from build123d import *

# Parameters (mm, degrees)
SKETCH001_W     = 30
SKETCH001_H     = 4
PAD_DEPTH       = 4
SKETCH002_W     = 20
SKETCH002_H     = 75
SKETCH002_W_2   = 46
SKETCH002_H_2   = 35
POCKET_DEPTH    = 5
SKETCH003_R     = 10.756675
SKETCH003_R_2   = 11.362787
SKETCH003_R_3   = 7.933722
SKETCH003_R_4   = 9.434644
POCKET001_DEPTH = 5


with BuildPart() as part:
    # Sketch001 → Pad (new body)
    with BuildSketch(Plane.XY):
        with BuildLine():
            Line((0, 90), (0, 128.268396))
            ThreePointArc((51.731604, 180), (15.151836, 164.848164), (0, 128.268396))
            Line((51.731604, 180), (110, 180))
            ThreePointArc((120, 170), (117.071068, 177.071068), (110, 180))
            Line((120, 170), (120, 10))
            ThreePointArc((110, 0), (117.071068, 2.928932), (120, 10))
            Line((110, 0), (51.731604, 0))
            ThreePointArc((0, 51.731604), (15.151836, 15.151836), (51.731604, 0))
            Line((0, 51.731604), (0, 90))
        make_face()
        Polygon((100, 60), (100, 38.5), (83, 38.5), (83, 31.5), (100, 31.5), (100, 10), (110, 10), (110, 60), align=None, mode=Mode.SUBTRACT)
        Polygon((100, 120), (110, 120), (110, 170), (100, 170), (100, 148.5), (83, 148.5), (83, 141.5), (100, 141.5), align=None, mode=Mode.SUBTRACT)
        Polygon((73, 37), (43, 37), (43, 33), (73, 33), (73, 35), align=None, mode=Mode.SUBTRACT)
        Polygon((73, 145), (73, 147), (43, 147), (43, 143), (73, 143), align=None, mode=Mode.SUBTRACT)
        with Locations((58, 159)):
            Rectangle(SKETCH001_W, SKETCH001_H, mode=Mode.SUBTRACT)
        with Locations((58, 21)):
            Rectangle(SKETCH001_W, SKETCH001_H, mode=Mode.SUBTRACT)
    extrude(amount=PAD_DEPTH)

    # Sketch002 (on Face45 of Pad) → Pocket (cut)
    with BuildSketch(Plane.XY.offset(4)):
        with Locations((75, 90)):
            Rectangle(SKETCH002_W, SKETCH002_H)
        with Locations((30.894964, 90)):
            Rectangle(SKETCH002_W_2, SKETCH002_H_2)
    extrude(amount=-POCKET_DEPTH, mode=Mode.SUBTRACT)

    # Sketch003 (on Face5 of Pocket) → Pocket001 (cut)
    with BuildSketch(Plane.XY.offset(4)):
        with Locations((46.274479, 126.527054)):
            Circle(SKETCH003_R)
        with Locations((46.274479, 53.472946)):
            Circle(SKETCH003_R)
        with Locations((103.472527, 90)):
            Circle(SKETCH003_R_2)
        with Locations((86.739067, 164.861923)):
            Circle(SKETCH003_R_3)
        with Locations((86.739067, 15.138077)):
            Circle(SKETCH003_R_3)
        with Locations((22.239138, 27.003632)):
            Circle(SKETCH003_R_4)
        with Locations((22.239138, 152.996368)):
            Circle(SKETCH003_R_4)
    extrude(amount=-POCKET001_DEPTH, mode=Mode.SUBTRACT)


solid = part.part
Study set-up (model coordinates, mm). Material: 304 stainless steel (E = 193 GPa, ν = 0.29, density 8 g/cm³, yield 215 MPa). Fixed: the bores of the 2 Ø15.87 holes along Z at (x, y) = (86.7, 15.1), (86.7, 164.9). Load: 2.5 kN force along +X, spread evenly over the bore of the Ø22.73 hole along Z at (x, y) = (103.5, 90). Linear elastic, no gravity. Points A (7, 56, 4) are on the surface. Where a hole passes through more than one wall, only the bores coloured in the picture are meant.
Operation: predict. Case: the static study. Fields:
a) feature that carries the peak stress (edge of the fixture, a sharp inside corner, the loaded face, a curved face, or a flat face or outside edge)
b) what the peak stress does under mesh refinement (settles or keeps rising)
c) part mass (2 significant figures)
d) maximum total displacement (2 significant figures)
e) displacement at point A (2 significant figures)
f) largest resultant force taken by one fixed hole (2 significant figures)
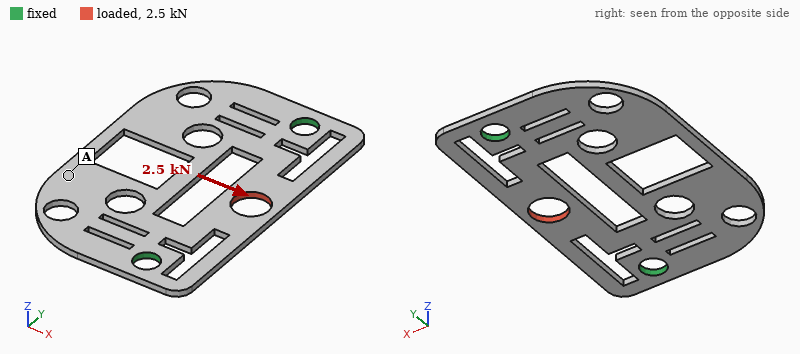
a sharp inside corner
keeps rising
430 g
31 µm
4.9 µm
1.3 kN
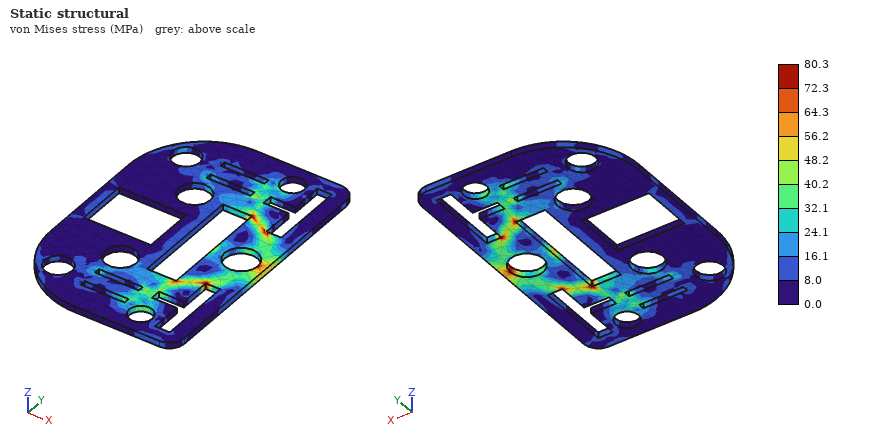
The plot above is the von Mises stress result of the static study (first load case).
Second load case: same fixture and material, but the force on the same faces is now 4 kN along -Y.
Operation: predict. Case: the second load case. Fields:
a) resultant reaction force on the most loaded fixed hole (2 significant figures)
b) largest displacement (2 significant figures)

2.1 kN
20 µm
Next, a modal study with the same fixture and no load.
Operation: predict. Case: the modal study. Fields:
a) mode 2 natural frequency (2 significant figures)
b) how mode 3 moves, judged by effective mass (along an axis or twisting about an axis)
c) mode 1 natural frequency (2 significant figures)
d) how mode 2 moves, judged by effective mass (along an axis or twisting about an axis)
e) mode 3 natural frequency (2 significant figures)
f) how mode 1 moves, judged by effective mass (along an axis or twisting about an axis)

720 Hz
twisting about X
360 Hz
along Z
770 Hz
along Z
